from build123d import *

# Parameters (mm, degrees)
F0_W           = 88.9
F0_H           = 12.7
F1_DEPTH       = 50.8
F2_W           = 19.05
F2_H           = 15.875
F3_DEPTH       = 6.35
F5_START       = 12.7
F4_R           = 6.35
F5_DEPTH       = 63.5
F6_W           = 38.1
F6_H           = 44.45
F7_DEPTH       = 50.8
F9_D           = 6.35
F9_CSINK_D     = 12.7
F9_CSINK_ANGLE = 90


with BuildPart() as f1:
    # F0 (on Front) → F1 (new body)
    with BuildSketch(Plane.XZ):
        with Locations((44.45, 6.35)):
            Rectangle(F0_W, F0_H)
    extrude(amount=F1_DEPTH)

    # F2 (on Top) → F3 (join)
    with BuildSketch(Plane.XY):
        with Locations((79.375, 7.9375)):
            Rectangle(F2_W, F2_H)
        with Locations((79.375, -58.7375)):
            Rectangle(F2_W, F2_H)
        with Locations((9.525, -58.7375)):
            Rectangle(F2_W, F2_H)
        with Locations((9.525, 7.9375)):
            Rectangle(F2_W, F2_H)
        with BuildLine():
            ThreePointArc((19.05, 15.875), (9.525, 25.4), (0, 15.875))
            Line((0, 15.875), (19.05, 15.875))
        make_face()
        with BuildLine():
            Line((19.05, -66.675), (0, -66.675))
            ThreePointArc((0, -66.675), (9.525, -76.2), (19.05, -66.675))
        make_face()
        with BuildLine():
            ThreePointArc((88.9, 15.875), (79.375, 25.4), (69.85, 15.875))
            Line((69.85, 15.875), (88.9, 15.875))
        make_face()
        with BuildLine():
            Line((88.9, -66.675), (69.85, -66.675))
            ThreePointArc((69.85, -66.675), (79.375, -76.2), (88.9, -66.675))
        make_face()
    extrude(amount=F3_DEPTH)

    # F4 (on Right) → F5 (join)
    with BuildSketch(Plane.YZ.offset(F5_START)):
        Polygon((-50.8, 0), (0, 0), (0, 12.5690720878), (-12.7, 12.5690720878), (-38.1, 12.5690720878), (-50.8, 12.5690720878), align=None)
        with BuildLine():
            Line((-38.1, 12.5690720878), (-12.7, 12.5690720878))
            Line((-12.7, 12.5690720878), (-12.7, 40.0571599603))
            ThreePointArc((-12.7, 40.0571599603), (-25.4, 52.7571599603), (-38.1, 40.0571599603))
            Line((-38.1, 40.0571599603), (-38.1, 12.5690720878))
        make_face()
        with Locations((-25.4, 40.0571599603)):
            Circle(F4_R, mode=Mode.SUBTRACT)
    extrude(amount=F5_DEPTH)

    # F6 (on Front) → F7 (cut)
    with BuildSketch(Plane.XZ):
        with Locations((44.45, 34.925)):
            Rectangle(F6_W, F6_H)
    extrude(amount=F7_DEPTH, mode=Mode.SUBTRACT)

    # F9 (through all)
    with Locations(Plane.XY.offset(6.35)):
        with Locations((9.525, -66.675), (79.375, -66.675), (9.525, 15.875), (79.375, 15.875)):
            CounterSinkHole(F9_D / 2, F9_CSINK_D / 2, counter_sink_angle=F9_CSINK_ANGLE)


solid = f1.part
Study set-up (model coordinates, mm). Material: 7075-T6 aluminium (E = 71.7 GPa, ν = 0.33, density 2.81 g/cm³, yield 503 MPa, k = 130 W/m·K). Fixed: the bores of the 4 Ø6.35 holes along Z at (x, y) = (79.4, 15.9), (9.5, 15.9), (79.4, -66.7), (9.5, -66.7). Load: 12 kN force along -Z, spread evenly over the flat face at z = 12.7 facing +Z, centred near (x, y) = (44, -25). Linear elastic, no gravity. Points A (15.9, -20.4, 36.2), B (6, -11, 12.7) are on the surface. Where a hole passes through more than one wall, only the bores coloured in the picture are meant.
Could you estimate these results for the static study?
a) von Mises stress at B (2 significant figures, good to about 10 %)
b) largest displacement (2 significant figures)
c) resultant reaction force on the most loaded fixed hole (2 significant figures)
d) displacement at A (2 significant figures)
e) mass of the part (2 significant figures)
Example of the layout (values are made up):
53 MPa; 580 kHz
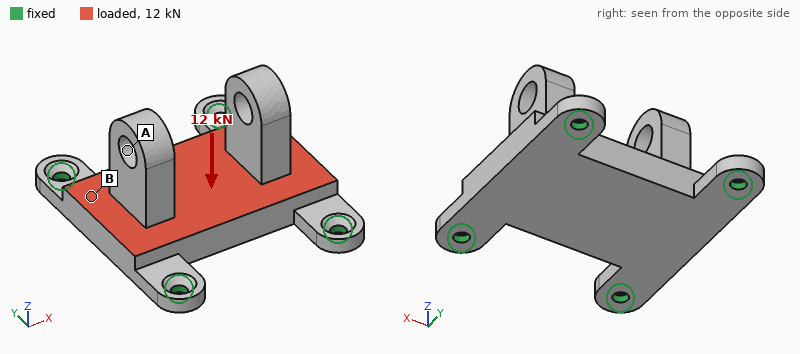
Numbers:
48 MPa; 0.16 mm; 4.9 kN; 0.13 mm; 250 g
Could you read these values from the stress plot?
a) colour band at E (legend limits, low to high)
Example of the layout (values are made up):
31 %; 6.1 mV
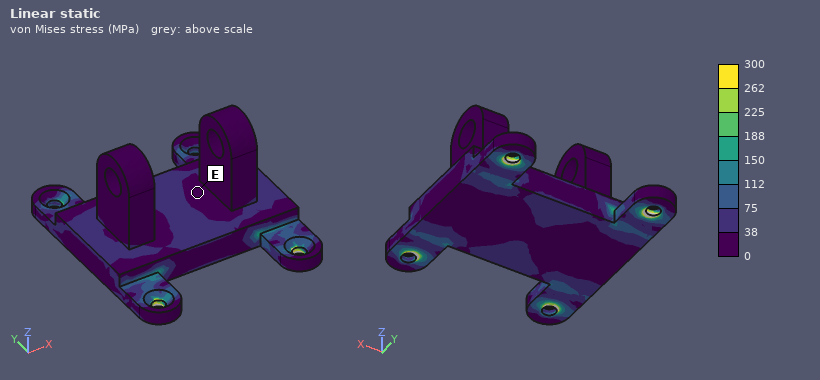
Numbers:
0 to 38 MPa
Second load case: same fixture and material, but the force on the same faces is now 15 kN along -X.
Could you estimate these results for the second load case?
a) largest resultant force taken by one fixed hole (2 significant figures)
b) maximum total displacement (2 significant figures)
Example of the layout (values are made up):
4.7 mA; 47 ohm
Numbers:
4.5 kN; 0.12 mm
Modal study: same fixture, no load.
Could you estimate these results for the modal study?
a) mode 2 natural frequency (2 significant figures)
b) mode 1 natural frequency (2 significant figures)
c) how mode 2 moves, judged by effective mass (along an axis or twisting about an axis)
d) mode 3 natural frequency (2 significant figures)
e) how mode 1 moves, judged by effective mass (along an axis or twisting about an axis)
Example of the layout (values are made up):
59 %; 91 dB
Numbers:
3600 Hz; 3100 Hz; along X; 4600 Hz; along Z
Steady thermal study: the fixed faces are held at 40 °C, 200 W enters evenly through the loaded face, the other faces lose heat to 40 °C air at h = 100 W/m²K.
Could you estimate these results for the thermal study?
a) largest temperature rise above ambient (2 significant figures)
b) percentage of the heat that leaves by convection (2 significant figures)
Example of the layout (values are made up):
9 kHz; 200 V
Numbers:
58 K; 36 %
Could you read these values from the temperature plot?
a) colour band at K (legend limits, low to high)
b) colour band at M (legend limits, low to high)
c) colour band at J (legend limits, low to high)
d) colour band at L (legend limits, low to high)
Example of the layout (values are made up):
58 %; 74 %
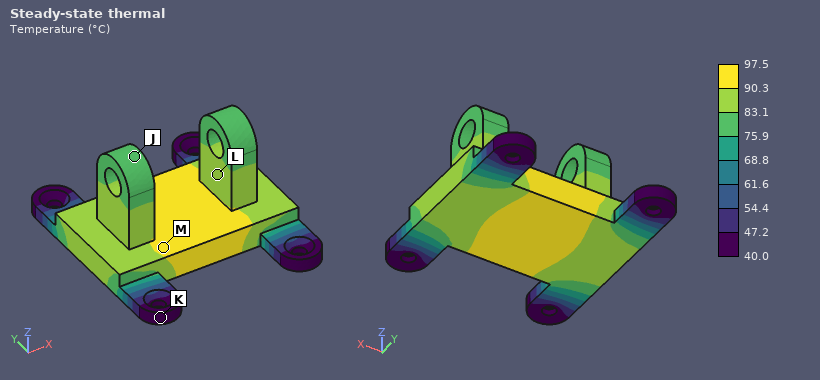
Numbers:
40.0 to 47.2 °C; 90.3 to 97.5 °C; 75.9 to 83.1 °C; 83.1 to 90.3 °C
